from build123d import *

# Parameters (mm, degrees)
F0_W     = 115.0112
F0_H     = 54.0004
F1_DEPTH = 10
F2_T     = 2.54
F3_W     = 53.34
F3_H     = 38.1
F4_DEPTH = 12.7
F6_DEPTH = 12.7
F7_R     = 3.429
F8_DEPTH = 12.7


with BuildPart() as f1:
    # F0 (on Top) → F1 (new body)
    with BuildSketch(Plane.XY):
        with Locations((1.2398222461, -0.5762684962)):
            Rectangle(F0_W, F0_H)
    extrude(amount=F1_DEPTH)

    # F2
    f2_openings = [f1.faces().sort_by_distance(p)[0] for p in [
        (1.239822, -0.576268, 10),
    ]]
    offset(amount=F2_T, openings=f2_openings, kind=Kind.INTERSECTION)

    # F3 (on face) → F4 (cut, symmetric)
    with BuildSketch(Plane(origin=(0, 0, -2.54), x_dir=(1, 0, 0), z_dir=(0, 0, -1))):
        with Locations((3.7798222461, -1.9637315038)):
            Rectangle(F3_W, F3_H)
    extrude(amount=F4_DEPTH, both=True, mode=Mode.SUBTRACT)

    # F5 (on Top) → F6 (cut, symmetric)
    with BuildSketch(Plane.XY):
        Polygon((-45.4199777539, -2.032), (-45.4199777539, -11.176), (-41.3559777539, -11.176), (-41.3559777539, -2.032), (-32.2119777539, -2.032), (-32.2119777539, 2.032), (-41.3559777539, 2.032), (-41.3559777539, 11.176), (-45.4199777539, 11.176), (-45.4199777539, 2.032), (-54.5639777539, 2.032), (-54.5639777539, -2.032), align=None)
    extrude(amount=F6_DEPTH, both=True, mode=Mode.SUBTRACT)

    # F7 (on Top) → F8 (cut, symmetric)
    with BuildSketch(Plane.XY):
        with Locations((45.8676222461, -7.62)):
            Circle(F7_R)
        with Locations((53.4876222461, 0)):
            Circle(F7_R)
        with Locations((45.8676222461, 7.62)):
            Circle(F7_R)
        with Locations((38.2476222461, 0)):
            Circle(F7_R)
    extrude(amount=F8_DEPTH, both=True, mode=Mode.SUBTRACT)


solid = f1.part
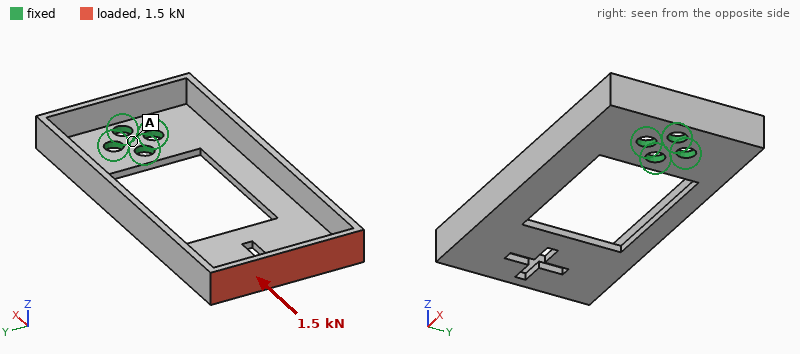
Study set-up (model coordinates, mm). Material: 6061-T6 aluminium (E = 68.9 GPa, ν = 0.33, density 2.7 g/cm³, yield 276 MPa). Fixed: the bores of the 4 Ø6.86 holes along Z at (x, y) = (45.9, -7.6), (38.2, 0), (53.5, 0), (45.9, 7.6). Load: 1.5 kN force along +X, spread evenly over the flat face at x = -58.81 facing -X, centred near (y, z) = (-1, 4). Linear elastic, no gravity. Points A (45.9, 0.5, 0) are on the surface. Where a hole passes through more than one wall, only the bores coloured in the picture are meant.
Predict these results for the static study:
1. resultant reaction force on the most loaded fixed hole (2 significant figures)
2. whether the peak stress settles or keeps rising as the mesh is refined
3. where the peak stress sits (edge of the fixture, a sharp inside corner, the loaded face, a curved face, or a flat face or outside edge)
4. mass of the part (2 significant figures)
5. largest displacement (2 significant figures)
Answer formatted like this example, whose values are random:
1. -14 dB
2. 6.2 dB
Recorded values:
1. 870 N
2. keeps rising
3. edge of the fixture
4. 56 g
5. 0.88 mm
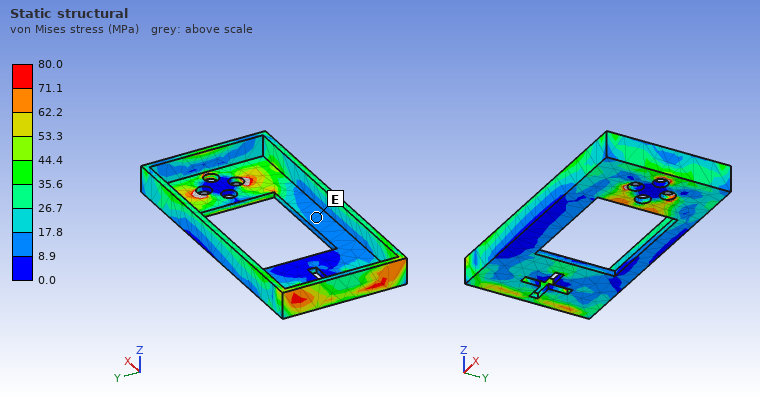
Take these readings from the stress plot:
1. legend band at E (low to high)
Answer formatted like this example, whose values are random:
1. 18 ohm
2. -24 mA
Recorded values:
1. 8.9 to 17.8 MPa
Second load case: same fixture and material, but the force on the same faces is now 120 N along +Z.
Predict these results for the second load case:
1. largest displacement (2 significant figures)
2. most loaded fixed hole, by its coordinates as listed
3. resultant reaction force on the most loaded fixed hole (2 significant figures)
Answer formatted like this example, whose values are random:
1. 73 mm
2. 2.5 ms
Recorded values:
1. 1.5 mm
2. (53.5, 0)
3. 640 N
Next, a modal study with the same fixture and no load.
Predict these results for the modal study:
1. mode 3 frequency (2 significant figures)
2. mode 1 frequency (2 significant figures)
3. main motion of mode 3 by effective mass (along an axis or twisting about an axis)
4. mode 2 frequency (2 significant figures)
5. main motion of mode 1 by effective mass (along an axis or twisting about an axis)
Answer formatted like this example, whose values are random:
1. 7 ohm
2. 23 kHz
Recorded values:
1. 1100 Hz
2. 330 Hz
3. along Y
4. 560 Hz
5. along Z
